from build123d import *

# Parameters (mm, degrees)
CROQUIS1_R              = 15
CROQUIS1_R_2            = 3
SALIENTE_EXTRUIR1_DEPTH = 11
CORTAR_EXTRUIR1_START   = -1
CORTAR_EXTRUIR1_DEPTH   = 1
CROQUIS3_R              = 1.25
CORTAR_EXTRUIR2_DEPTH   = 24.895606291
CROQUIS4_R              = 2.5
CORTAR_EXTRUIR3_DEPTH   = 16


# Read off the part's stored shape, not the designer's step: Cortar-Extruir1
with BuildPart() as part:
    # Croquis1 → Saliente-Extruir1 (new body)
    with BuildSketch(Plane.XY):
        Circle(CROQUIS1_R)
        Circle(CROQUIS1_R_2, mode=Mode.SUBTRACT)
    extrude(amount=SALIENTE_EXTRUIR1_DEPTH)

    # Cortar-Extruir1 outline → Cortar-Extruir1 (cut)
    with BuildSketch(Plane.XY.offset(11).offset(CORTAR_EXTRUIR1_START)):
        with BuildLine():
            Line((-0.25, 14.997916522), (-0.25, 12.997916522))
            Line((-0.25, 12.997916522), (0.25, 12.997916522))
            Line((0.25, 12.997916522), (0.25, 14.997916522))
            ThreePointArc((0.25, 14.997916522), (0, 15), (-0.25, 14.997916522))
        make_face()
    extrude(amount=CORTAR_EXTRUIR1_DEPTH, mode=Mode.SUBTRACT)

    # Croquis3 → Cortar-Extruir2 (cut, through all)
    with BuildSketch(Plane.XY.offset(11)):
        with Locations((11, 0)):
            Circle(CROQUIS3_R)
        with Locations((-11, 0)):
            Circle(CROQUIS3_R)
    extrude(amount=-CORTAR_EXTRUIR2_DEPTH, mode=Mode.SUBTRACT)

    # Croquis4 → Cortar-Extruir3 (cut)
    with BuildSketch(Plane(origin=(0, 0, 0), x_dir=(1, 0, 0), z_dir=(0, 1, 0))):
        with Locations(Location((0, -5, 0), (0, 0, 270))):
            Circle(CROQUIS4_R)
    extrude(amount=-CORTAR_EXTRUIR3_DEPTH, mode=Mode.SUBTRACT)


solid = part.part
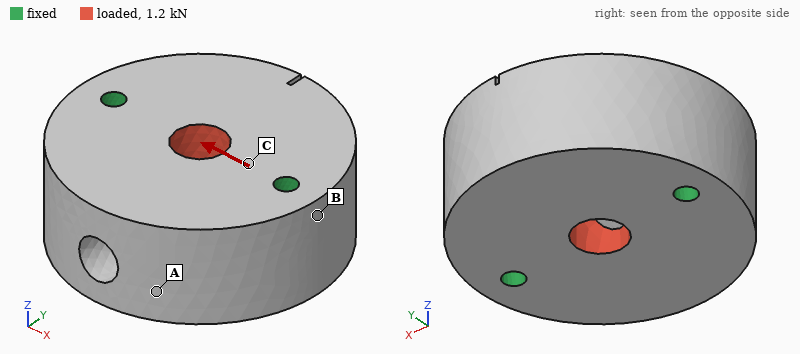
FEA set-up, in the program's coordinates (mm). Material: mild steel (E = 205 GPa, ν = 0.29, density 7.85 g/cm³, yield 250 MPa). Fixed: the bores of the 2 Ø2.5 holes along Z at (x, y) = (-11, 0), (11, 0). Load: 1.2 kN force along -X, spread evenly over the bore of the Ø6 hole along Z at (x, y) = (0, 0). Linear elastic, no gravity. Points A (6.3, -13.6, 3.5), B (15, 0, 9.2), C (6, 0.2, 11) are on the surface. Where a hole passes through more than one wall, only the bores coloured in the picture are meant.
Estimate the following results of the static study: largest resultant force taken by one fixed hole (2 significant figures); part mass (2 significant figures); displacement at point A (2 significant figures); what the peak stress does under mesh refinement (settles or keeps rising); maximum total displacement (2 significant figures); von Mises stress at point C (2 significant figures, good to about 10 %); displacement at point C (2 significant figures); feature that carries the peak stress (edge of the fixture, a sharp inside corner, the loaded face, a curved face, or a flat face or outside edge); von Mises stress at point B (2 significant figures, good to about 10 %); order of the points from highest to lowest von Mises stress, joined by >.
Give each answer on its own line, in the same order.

600 N
56 g
0.14 µm
keeps rising
0.35 µm
8.1 MPa
0.18 µm
edge of the fixture
3.9 MPa
C > B > A
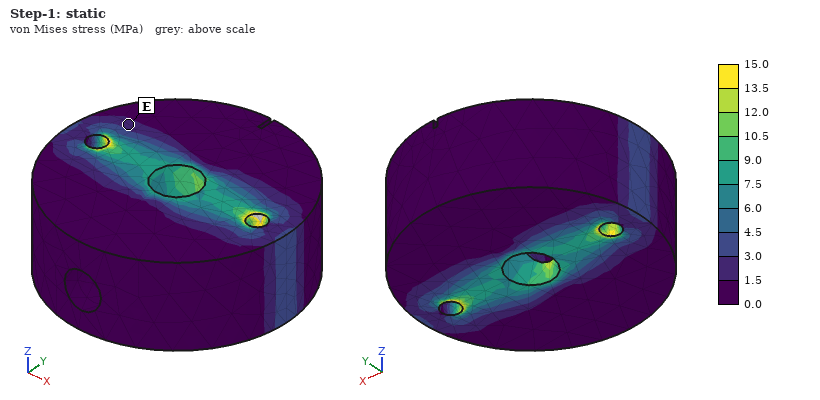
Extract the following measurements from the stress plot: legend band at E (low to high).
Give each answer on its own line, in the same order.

1.5 to 3.0 MPa
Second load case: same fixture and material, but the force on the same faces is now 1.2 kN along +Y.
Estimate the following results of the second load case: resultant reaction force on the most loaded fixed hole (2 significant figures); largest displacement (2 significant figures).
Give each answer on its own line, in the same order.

600 N
0.49 µm
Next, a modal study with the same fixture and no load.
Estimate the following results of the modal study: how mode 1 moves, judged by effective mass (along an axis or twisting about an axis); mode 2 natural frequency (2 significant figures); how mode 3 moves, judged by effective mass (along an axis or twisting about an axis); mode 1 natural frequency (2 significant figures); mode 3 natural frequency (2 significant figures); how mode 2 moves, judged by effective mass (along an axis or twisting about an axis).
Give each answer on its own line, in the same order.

twisting about X
32 kHz
twisting about Z
26 kHz
49 kHz
along Z
